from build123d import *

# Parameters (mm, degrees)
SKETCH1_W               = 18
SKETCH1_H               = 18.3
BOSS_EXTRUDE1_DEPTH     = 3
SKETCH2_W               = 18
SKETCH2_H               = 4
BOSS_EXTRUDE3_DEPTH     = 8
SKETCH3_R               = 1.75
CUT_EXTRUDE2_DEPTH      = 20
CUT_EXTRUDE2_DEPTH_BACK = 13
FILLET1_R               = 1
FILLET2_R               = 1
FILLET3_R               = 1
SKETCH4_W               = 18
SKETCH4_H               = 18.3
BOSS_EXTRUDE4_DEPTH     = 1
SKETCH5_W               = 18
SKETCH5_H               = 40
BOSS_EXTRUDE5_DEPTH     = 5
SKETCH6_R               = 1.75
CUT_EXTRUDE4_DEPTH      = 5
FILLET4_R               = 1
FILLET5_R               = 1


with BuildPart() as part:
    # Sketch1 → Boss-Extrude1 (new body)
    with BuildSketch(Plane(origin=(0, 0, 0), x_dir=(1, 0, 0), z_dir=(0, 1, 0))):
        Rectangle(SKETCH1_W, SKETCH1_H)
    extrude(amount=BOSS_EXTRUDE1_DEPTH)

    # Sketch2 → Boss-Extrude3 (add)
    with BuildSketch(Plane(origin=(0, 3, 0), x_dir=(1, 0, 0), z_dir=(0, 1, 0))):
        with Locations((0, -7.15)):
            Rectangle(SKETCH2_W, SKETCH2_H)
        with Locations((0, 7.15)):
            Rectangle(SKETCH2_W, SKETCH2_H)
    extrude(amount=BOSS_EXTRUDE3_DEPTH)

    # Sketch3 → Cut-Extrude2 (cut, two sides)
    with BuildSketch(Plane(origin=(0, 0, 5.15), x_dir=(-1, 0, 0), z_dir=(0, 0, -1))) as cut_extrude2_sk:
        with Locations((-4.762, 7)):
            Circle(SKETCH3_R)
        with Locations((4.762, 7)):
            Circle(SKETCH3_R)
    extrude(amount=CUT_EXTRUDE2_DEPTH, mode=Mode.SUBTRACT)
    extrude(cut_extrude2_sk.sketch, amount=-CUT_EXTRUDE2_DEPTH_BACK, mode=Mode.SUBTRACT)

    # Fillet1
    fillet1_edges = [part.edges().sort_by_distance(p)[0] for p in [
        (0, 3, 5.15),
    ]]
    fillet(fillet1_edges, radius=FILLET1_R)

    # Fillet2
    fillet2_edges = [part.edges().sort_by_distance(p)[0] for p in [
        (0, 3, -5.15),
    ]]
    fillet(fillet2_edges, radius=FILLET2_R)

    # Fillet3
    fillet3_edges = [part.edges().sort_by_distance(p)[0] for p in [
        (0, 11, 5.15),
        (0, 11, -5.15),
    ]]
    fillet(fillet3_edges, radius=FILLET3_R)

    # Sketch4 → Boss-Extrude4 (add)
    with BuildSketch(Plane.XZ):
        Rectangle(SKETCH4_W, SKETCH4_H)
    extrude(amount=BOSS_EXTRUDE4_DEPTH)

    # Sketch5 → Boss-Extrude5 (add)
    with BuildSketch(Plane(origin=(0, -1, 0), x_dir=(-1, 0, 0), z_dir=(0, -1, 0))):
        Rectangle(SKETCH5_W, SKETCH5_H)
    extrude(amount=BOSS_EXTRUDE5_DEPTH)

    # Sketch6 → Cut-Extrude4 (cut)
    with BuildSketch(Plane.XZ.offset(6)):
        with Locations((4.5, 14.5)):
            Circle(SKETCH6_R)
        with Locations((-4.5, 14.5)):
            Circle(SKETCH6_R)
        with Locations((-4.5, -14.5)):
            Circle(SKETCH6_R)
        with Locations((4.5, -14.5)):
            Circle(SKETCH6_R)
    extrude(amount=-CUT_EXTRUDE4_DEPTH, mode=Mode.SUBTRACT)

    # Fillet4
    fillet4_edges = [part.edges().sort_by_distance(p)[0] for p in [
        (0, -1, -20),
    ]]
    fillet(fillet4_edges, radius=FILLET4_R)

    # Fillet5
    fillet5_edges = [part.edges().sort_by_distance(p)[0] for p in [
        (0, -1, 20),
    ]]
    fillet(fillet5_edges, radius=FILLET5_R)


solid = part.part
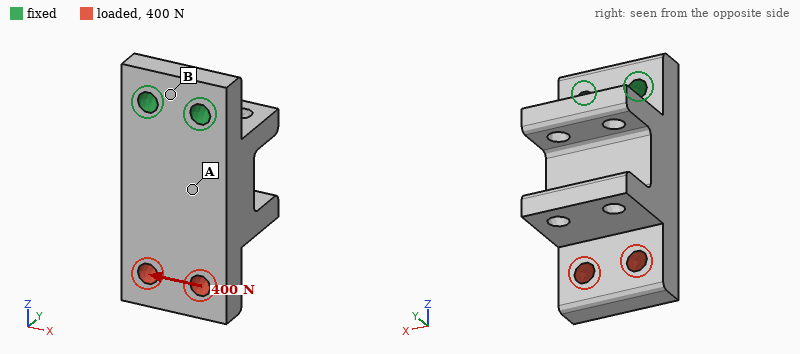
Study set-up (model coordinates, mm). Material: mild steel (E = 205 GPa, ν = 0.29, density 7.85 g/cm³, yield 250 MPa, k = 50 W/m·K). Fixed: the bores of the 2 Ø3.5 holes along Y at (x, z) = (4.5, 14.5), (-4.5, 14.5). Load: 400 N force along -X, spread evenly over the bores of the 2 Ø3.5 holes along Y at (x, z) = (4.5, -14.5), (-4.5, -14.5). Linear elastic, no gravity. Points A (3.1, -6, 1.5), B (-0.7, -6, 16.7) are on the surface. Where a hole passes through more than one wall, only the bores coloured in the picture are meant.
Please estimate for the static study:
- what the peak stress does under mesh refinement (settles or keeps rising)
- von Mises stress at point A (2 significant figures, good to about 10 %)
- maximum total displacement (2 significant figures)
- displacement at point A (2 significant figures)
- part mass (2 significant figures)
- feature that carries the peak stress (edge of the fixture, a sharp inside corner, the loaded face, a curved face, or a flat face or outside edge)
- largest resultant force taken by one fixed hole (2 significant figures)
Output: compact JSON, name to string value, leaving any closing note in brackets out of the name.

{"what the peak stress does under mesh refinement": "keeps rising", "von Mises stress at point A": "15 MPa", "maximum total displacement": "10 µm", "displacement at point A": "2.8 µm", "part mass": "45 g", "feature that carries the peak stress": "edge of the fixture", "largest resultant force taken by one fixed hole": "1.0 kN"}
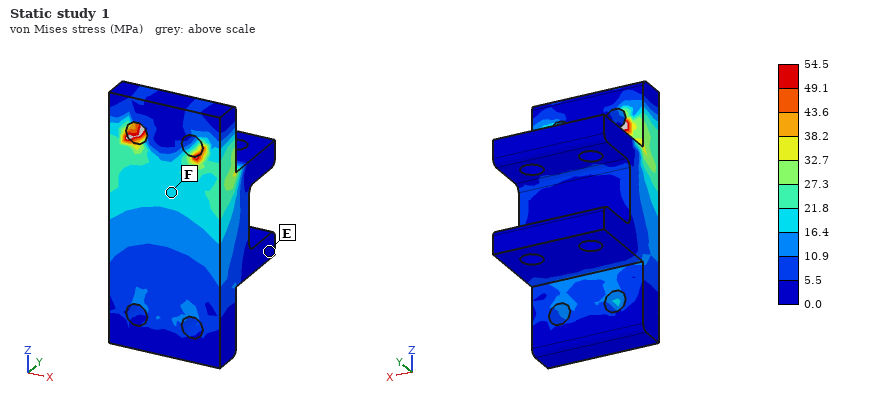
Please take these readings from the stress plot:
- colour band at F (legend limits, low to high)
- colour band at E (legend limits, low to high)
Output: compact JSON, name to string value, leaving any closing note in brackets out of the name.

{"colour band at F": "16.4 to 21.8 MPa", "colour band at E": "0.0 to 5.5 MPa"}
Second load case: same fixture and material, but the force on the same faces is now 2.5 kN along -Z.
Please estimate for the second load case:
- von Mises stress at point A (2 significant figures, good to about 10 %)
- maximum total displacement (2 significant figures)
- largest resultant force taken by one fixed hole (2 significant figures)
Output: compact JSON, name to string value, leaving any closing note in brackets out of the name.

{"von Mises stress at point A": "36 MPa", "maximum total displacement": "8.7 µm", "largest resultant force taken by one fixed hole": "1.3 kN"}
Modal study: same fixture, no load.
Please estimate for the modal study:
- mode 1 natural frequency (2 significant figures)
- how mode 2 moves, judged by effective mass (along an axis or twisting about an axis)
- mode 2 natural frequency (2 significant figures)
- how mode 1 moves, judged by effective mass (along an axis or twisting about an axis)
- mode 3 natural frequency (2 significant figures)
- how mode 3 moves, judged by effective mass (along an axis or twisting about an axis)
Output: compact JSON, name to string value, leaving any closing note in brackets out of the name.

{"mode 1 natural frequency": "3600 Hz", "how mode 2 moves, judged by effective mass": "along X", "mode 2 natural frequency": "9500 Hz", "how mode 1 moves, judged by effective mass": "along Y", "mode 3 natural frequency": "13 kHz", "how mode 3 moves, judged by effective mass": "twisting about Z"}
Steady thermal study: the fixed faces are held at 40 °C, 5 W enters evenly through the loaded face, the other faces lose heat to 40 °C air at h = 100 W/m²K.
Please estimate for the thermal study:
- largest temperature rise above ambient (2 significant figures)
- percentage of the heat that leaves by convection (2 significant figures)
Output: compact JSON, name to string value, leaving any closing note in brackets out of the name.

{"largest temperature rise above ambient": "19 K", "percentage of the heat that leaves by convection": "44 %"}
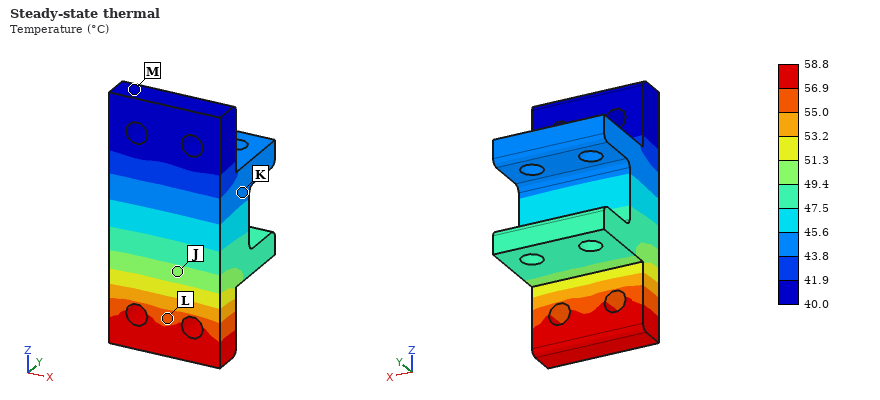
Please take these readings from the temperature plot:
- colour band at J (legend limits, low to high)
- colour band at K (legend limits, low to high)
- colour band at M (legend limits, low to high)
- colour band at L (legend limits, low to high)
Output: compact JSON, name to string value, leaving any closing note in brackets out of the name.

{"colour band at J": "49.4 to 51.3 °C", "colour band at K": "43.8 to 45.6 °C", "colour band at M": "40.0 to 41.9 °C", "colour band at L": "55.0 to 56.9 °C"}
